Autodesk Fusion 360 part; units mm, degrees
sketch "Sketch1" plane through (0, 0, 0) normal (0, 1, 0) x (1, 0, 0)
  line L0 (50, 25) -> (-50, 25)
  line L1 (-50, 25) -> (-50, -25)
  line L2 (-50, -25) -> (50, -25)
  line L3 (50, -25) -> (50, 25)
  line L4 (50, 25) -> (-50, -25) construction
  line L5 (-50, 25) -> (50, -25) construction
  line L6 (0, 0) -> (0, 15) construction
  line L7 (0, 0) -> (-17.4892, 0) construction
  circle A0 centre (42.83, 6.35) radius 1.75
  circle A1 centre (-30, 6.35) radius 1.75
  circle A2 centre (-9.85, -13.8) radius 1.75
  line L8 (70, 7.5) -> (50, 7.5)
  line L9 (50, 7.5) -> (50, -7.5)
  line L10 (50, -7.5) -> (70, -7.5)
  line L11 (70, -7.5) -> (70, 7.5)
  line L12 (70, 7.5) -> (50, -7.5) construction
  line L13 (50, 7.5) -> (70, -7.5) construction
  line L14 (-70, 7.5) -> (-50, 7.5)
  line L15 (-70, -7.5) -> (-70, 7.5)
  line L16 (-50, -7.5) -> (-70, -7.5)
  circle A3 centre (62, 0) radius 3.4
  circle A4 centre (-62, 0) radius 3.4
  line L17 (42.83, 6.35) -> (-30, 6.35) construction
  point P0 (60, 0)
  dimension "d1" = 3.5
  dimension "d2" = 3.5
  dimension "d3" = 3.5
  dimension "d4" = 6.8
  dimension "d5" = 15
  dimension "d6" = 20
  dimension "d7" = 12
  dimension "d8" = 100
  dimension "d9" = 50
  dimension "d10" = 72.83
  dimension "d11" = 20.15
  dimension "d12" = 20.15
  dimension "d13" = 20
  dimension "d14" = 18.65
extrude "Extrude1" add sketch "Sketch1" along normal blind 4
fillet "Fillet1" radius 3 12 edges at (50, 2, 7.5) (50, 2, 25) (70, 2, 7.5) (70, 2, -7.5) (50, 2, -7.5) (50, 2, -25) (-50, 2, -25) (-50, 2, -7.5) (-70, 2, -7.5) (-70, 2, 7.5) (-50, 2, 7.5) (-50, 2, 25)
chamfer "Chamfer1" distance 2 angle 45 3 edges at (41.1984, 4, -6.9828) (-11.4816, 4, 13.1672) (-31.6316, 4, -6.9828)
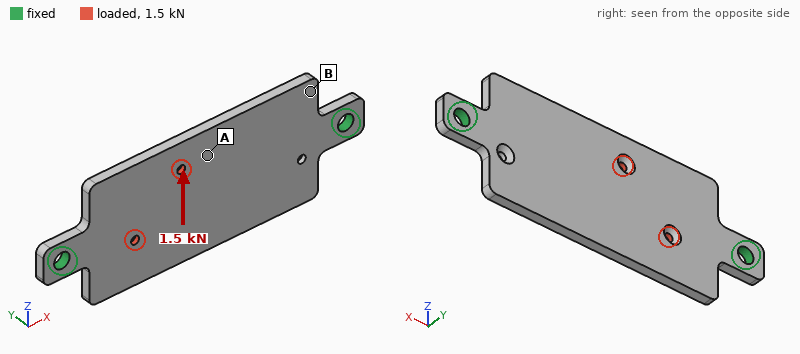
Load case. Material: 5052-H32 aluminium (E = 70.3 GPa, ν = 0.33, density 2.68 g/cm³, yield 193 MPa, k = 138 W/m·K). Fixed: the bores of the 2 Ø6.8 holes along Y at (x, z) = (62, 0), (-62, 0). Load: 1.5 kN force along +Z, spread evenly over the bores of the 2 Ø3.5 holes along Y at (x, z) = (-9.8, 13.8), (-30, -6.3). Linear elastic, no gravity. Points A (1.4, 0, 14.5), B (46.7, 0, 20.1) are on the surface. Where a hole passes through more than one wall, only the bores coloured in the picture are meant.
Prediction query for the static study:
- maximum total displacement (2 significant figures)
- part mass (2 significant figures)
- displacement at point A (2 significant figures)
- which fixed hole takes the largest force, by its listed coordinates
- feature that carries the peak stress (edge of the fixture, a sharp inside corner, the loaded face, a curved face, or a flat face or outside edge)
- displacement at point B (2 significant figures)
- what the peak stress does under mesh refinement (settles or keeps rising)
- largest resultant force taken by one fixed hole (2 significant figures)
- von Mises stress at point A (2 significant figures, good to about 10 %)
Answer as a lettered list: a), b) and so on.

a) 66 µm
b) 59 g
c) 42 µm
d) (-62, 0)
e) edge of the fixture
f) 25 µm
g) keeps rising
h) 1.0 kN
i) 11 MPa
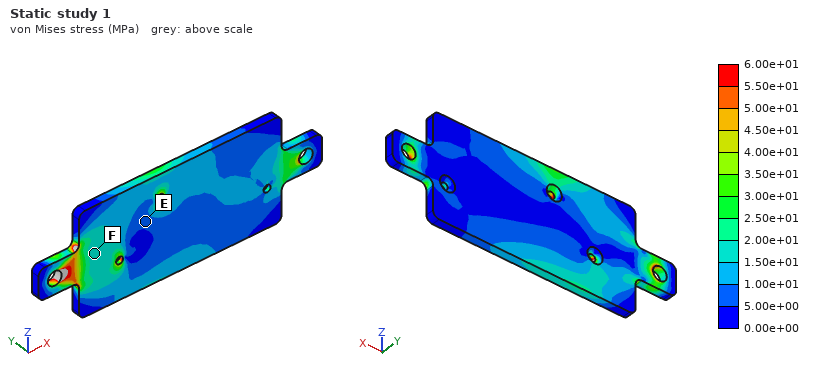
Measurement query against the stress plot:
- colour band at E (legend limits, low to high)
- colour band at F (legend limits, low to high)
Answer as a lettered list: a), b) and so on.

a) 5.00e+00 to 1.00e+01 MPa
b) 1.50e+01 to 2.00e+01 MPa
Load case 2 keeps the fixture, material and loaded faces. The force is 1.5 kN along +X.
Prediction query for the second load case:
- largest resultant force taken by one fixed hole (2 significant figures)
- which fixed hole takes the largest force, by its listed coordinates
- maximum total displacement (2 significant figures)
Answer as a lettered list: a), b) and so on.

a) 910 N
b) (-62, 0)
c) 22 µm
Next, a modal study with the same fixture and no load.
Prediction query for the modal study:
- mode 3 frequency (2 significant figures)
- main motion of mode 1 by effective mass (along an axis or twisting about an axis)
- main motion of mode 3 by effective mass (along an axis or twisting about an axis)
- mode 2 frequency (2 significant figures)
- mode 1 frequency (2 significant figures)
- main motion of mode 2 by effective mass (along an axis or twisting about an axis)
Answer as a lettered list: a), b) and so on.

a) 3100 Hz
b) along Y
c) twisting about Z
d) 1400 Hz
e) 1100 Hz
f) twisting about X
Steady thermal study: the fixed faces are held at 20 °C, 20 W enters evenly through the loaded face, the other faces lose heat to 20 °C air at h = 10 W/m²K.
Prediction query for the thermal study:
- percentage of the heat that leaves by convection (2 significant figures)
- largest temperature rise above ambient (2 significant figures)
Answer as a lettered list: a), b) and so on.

a) 12 %
b) 35 K
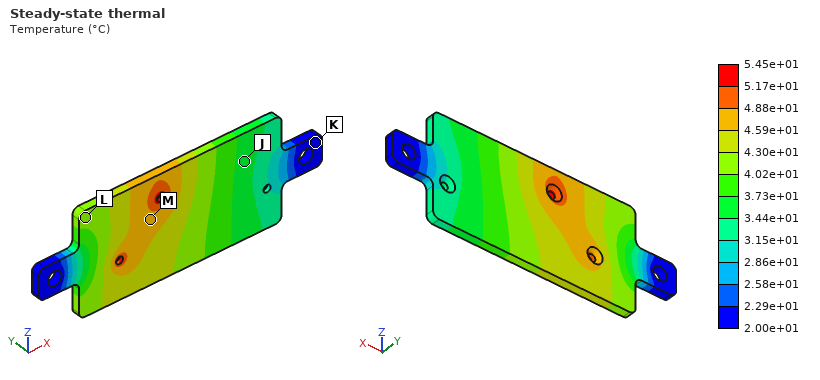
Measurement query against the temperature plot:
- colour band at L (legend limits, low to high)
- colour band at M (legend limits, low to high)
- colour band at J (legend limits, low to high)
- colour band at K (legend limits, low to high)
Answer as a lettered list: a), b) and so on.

a) 4.02e+01 to 4.30e+01 °C
b) 4.59e+01 to 4.88e+01 °C
c) 3.44e+01 to 3.73e+01 °C
d) 2.00e+01 to 2.29e+01 °C
